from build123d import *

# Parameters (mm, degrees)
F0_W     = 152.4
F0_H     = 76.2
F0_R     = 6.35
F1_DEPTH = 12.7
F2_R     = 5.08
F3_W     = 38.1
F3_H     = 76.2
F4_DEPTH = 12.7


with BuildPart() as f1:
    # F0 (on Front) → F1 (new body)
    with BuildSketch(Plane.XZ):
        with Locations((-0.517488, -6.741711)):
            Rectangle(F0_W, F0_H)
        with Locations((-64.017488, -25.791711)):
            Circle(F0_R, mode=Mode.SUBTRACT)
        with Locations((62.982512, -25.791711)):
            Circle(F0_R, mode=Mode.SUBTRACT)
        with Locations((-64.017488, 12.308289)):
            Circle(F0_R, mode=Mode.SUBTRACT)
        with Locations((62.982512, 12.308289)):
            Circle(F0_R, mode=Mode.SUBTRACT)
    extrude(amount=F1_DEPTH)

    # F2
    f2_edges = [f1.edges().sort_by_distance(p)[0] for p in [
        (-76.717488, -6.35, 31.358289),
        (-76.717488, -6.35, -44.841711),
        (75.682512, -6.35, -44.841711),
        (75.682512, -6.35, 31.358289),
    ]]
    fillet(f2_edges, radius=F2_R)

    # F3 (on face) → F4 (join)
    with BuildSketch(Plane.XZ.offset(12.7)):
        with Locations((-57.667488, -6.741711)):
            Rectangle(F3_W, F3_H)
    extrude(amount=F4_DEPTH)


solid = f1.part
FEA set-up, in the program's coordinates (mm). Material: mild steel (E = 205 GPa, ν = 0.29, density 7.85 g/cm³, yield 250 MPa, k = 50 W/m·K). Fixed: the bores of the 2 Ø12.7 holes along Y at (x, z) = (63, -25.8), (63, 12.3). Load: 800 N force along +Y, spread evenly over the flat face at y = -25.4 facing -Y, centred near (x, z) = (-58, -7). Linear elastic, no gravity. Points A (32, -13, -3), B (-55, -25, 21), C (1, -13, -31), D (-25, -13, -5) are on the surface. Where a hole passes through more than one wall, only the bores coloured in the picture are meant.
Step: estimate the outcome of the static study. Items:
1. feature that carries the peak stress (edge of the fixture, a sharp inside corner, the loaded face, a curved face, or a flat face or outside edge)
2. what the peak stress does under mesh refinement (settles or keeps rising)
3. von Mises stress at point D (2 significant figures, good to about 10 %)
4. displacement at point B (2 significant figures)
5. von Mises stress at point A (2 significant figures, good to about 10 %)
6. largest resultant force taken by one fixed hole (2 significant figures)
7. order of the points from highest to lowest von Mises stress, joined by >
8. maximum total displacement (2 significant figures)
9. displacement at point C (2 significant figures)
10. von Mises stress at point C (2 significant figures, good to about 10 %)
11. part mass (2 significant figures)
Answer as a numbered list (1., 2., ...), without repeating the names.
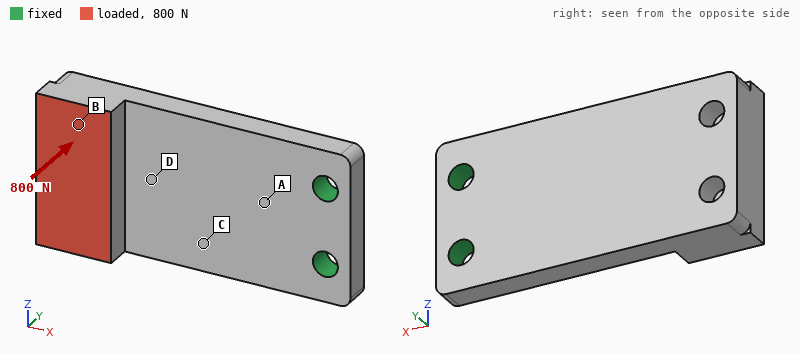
1. edge of the fixture
2. keeps rising
3. 13 MPa
4. 0.16 mm
5. 32 MPa
6. 400 N
7. A > C > D > B
8. 0.20 mm
9. 0.052 mm
10. 23 MPa
11. 1.4 kg
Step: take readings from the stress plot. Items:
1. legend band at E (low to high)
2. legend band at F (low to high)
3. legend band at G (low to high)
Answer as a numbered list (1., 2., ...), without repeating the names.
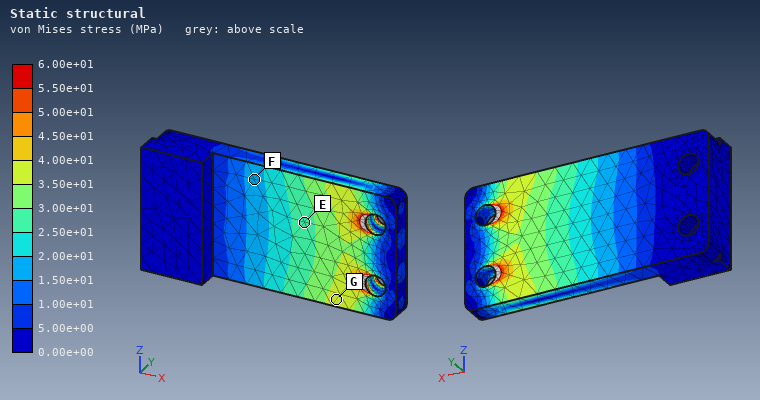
1. 2.50e+01 to 3.00e+01 MPa
2. 1.50e+01 to 2.00e+01 MPa
3. 3.50e+01 to 4.00e+01 MPa
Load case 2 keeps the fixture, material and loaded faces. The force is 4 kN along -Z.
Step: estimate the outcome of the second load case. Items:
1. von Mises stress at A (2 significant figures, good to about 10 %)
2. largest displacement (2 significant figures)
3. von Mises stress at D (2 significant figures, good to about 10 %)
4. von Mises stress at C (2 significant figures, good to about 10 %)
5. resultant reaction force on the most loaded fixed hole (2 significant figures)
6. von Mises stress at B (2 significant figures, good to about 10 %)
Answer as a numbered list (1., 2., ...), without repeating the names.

1. 42 MPa
2. 94 µm
3. 34 MPa
4. 40 MPa
5. 10 kN
6. 7.6 MPa
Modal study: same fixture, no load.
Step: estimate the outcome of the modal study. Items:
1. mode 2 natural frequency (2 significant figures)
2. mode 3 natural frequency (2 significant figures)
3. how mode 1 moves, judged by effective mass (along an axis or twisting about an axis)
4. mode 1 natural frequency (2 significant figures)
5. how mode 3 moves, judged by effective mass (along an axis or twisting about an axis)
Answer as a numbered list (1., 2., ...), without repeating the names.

1. 1600 Hz
2. 2100 Hz
3. along Y
4. 430 Hz
5. along Z
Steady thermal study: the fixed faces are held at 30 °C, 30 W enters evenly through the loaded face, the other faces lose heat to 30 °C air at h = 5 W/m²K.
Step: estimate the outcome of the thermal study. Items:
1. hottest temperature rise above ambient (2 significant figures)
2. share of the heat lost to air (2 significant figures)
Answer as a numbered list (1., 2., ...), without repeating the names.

1. 63 K
2. 16 %
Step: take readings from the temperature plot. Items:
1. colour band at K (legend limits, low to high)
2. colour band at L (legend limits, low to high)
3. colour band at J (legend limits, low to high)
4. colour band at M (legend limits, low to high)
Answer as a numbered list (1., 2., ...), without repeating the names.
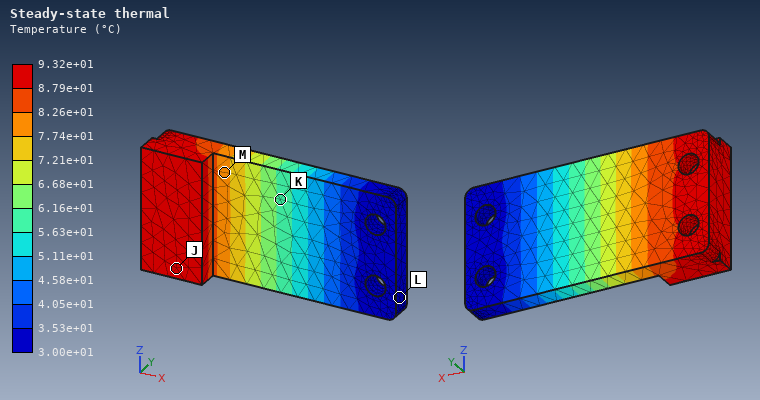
1. 5.63e+01 to 6.16e+01 °C
2. 3.00e+01 to 3.53e+01 °C
3. 8.79e+01 to 9.32e+01 °C
4. 7.74e+01 to 8.26e+01 °C
